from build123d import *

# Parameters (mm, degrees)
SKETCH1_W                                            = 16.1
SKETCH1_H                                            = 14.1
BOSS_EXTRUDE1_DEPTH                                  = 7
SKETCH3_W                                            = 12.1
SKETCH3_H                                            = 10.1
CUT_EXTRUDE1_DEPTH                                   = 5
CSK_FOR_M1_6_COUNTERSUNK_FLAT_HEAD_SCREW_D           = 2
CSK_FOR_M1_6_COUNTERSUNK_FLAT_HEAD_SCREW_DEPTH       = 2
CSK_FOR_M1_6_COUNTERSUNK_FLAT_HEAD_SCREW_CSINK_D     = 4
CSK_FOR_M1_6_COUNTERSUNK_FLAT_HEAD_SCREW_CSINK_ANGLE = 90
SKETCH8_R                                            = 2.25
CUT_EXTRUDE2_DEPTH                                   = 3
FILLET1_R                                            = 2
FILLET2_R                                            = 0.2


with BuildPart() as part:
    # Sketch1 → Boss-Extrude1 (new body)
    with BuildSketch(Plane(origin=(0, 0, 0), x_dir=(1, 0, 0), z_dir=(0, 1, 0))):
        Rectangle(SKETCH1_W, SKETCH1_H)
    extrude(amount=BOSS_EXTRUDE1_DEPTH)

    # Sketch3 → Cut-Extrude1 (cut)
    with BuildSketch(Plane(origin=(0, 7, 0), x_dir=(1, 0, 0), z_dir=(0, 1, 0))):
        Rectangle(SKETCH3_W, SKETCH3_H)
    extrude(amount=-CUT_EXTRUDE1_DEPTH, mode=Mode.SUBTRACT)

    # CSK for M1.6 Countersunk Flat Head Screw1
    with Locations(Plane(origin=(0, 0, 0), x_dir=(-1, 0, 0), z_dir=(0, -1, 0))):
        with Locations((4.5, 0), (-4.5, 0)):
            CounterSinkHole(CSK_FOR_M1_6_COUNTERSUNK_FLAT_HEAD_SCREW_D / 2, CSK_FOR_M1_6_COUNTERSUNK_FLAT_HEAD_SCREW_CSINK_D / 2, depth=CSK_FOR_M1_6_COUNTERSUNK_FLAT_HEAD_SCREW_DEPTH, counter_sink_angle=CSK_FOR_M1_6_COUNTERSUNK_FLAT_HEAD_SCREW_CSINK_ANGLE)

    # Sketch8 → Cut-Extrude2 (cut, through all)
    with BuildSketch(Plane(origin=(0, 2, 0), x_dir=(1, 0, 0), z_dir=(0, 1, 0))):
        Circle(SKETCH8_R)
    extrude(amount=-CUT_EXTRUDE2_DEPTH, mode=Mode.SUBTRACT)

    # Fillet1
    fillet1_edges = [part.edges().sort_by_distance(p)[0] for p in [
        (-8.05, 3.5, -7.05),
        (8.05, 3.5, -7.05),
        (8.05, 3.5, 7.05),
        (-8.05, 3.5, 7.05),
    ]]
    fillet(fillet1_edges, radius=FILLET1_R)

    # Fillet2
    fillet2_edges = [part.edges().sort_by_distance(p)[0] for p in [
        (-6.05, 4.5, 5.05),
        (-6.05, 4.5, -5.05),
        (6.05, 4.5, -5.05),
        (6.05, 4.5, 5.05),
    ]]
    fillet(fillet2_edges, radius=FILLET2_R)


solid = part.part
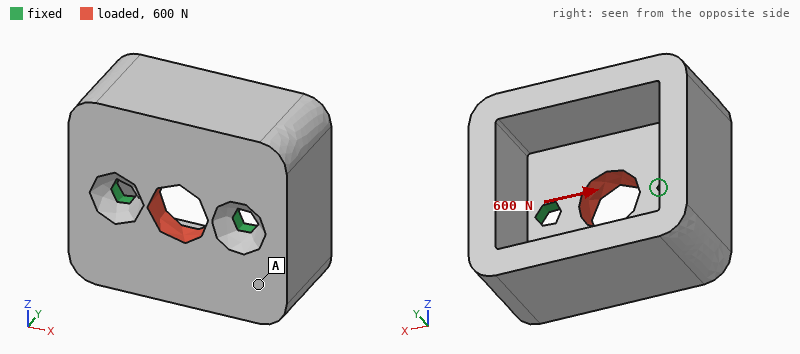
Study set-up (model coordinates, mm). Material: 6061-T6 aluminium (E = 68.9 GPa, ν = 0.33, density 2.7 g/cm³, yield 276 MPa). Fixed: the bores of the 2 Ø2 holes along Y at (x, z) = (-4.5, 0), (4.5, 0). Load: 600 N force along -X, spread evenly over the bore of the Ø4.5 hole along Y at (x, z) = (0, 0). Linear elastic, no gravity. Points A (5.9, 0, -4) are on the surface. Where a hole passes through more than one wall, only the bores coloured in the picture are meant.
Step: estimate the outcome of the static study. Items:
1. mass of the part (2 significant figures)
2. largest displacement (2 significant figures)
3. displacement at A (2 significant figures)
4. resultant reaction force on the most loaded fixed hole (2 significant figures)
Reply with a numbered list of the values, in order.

1. 2.4 g
2. 2.2 µm
3. 1.2 µm
4. 300 N
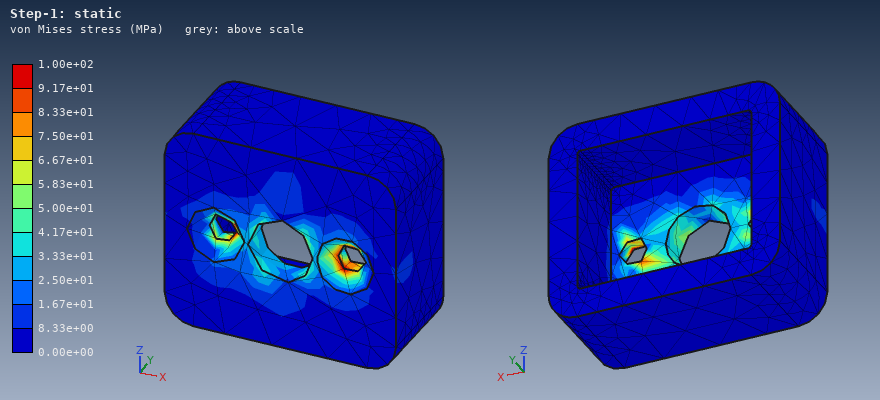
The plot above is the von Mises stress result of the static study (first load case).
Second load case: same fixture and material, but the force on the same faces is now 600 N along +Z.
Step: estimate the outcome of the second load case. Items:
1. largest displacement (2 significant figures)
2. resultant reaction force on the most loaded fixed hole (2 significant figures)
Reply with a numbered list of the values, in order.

1. 5.9 µm
2. 300 N
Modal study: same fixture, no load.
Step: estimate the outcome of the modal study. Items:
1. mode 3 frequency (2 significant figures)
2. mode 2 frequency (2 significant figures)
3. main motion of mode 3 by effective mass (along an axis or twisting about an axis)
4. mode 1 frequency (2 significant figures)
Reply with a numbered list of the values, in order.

1. 28 kHz
2. 24 kHz
3. along X
4. 11 kHz
